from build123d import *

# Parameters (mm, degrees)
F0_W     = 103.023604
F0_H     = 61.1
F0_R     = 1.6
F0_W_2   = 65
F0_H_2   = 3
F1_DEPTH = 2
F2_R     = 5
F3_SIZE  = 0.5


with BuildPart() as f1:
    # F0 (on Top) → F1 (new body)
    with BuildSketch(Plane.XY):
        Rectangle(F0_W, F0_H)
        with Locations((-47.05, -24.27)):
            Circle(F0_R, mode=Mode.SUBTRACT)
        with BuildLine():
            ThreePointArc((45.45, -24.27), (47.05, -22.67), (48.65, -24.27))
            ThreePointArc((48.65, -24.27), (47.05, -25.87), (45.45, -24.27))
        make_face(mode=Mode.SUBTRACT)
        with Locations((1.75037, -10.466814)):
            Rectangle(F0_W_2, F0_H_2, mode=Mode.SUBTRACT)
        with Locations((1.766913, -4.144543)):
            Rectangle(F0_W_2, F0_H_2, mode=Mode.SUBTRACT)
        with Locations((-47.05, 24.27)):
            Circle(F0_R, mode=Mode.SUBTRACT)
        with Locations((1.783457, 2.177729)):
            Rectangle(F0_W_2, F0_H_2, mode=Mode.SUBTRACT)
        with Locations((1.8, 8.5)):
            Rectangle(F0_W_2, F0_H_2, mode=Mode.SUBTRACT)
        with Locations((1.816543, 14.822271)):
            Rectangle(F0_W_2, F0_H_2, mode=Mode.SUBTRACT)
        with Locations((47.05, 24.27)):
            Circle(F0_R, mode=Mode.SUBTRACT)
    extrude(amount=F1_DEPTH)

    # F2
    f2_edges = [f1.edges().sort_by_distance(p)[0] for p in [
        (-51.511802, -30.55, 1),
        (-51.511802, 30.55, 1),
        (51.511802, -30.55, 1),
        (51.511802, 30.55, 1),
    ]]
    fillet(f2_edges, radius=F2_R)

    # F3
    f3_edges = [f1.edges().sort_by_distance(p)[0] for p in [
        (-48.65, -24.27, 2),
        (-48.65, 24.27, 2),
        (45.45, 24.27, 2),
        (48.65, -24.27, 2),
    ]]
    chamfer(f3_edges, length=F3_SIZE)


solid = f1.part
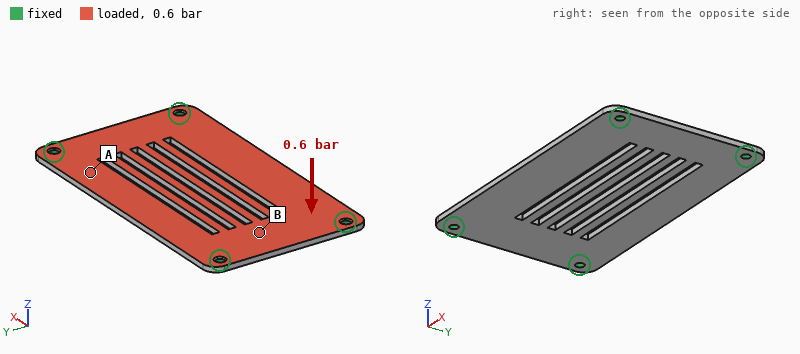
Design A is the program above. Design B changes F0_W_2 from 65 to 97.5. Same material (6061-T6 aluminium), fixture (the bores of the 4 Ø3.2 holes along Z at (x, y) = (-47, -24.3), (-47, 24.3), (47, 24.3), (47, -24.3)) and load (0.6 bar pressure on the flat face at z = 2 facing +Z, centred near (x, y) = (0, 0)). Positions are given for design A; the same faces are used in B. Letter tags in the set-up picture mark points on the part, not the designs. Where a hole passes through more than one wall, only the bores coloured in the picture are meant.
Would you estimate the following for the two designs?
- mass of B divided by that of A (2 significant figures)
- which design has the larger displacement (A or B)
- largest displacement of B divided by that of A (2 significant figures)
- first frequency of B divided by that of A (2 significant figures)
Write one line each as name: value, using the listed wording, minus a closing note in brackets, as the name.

mass of B divided by that of A: 0.91
which design has the larger displacement: B
largest displacement of B divided by that of A: 2.7
first frequency of B divided by that of A: 0.59
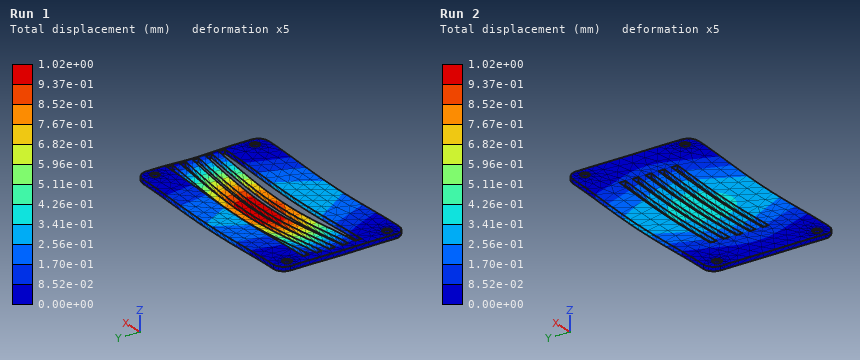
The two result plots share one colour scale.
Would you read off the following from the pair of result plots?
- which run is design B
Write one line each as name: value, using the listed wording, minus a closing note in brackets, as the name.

which run is design B: Run 1
